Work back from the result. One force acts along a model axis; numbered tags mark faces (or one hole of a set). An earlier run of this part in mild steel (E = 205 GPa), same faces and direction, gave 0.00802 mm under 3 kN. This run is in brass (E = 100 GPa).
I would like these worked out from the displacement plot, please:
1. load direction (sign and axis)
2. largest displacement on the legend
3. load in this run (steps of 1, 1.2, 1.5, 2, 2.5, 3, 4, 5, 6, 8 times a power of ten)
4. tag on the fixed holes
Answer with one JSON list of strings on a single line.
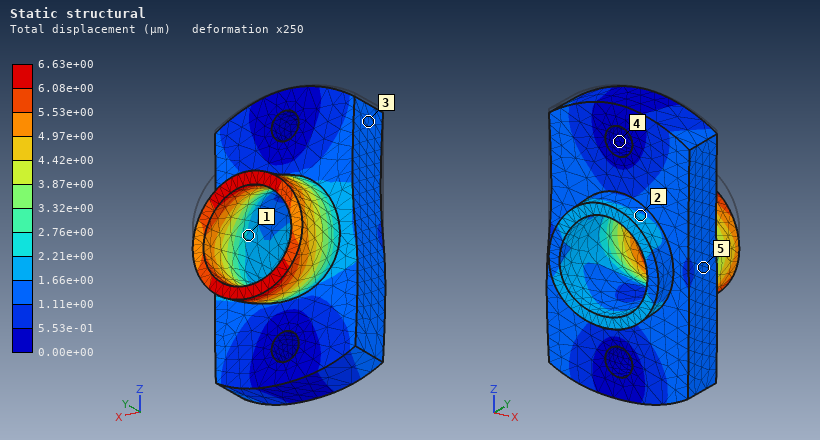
["-Z", "6.63e+00 µm", "1.2 kN", "4"]
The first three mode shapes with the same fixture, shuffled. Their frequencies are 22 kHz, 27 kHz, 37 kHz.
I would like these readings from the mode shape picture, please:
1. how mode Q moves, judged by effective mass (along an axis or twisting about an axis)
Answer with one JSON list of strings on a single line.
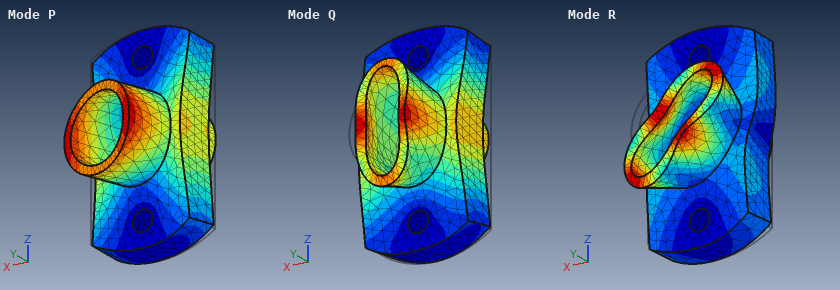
["along Y"]
